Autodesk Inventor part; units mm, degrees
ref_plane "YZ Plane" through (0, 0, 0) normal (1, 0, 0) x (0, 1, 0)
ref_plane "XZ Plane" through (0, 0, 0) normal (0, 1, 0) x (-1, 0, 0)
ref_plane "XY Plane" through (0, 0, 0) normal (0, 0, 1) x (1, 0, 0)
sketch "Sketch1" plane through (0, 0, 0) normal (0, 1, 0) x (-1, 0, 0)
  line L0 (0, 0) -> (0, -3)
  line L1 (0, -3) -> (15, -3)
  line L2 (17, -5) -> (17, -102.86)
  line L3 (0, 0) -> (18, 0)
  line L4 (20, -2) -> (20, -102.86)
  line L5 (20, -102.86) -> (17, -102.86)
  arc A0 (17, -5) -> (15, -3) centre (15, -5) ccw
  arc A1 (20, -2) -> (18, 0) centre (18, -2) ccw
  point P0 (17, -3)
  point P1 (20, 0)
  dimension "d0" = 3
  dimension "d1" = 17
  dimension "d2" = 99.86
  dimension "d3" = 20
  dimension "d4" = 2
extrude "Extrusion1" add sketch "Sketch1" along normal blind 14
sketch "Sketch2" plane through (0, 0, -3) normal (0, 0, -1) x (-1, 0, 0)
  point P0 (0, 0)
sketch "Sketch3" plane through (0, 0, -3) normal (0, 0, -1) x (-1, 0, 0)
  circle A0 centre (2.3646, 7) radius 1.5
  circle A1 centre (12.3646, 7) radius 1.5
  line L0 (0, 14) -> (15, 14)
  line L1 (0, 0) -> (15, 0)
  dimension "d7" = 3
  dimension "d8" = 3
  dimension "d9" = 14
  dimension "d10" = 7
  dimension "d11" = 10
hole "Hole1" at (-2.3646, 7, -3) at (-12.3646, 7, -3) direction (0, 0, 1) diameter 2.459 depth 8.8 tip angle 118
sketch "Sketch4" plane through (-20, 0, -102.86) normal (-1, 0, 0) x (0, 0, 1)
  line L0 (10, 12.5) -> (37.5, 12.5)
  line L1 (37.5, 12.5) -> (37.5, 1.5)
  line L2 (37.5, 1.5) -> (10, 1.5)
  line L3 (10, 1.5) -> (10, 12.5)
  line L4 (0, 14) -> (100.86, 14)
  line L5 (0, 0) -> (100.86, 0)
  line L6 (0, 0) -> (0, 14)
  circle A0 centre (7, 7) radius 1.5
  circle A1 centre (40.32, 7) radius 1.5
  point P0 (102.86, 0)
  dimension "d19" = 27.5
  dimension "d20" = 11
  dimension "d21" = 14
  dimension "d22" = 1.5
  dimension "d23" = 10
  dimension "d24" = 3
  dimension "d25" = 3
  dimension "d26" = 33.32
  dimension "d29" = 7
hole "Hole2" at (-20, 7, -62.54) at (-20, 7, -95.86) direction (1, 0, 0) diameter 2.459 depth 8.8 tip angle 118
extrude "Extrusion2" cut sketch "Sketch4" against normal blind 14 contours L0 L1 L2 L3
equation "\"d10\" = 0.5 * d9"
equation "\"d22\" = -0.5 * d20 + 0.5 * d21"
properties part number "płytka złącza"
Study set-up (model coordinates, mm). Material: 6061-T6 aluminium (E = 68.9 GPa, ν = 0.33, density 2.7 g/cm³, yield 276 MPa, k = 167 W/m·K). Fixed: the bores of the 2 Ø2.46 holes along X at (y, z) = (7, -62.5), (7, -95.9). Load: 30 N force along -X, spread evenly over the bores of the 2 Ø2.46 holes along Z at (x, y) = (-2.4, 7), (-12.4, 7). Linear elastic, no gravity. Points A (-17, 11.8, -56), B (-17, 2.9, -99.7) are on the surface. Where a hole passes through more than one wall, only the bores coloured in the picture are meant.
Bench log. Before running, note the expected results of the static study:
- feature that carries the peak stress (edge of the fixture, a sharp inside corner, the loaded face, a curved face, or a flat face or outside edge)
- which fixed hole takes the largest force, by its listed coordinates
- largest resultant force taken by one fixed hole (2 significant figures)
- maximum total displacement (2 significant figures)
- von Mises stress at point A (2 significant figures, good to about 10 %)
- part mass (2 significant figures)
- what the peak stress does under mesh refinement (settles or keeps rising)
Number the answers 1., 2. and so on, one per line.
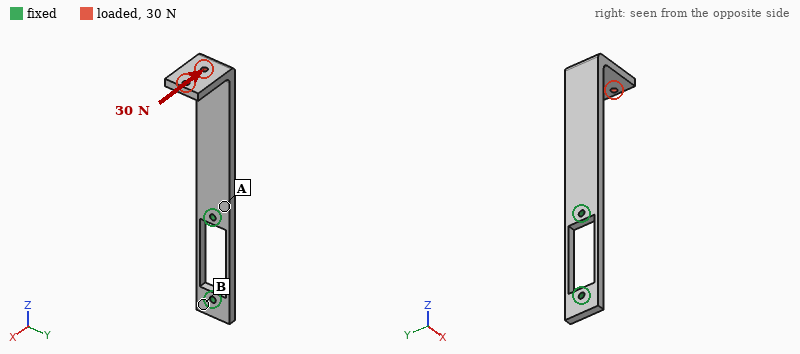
1. edge of the fixture
2. (7, -62.5)
3. 34 N
4. 1.2 mm
5. 75 MPa
6. 11 g
7. keeps rising
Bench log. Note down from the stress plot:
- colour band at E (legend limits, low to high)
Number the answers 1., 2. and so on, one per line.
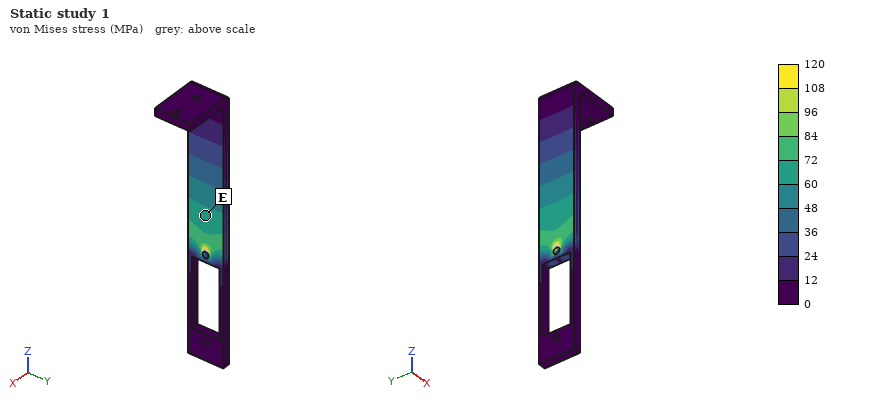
1. 60 to 72 MPa
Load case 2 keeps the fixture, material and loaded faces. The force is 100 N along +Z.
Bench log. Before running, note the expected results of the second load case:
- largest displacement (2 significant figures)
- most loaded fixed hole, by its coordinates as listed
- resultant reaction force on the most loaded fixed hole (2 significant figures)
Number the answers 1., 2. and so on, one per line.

1. 1.2 mm
2. (7, -62.5)
3. 95 N
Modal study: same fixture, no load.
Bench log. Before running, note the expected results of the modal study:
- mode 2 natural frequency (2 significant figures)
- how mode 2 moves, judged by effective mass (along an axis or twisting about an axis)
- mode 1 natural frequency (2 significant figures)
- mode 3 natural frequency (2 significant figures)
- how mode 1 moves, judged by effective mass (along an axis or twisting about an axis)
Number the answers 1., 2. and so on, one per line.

1. 1200 Hz
2. along Y
3. 430 Hz
4. 2500 Hz
5. along X
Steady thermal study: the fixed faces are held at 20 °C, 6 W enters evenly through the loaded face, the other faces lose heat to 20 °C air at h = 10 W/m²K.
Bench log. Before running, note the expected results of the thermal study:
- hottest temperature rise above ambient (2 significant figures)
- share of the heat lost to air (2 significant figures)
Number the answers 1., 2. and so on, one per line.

1. 57 K
2. 14 %
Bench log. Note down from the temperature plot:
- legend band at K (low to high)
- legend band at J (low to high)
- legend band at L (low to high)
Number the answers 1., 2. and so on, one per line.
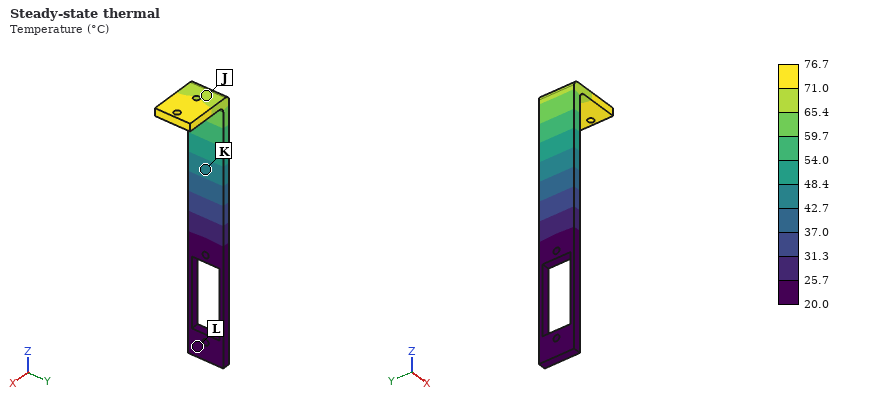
1. 42.7 to 48.4 °C
2. 65.4 to 71.0 °C
3. 20.0 to 25.7 °C
